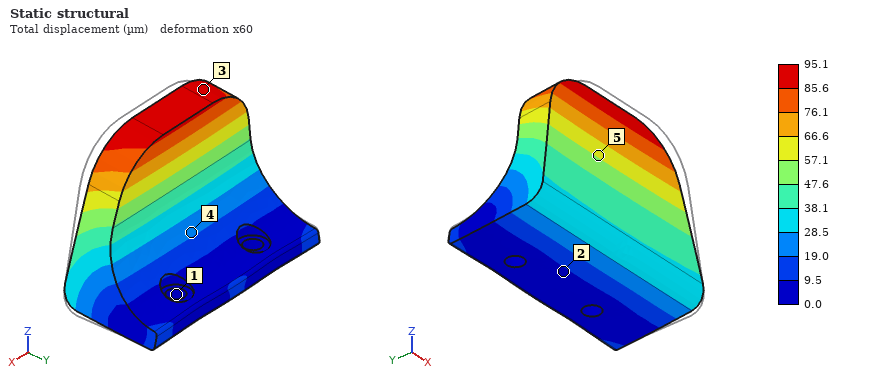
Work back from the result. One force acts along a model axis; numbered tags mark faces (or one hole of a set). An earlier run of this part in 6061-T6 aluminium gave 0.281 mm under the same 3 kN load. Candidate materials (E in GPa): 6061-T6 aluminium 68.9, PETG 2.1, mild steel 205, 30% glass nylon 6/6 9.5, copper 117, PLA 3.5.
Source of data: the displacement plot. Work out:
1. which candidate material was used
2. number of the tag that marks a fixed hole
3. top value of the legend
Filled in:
mild steel
1
95.1 µm
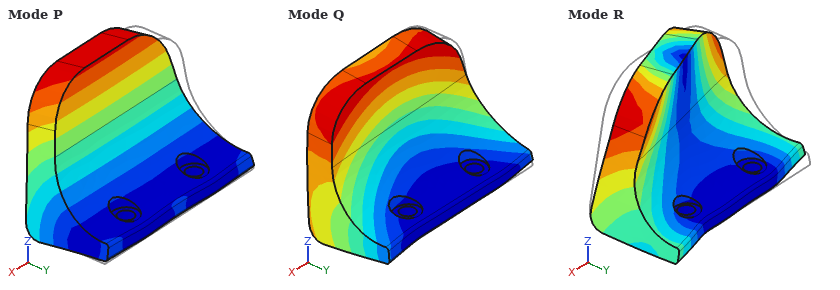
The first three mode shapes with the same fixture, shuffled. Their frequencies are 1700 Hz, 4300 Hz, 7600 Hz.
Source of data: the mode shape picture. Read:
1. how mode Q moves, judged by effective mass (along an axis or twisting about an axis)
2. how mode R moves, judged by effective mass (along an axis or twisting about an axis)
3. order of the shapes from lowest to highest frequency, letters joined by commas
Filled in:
along X
along X
P, Q, R
